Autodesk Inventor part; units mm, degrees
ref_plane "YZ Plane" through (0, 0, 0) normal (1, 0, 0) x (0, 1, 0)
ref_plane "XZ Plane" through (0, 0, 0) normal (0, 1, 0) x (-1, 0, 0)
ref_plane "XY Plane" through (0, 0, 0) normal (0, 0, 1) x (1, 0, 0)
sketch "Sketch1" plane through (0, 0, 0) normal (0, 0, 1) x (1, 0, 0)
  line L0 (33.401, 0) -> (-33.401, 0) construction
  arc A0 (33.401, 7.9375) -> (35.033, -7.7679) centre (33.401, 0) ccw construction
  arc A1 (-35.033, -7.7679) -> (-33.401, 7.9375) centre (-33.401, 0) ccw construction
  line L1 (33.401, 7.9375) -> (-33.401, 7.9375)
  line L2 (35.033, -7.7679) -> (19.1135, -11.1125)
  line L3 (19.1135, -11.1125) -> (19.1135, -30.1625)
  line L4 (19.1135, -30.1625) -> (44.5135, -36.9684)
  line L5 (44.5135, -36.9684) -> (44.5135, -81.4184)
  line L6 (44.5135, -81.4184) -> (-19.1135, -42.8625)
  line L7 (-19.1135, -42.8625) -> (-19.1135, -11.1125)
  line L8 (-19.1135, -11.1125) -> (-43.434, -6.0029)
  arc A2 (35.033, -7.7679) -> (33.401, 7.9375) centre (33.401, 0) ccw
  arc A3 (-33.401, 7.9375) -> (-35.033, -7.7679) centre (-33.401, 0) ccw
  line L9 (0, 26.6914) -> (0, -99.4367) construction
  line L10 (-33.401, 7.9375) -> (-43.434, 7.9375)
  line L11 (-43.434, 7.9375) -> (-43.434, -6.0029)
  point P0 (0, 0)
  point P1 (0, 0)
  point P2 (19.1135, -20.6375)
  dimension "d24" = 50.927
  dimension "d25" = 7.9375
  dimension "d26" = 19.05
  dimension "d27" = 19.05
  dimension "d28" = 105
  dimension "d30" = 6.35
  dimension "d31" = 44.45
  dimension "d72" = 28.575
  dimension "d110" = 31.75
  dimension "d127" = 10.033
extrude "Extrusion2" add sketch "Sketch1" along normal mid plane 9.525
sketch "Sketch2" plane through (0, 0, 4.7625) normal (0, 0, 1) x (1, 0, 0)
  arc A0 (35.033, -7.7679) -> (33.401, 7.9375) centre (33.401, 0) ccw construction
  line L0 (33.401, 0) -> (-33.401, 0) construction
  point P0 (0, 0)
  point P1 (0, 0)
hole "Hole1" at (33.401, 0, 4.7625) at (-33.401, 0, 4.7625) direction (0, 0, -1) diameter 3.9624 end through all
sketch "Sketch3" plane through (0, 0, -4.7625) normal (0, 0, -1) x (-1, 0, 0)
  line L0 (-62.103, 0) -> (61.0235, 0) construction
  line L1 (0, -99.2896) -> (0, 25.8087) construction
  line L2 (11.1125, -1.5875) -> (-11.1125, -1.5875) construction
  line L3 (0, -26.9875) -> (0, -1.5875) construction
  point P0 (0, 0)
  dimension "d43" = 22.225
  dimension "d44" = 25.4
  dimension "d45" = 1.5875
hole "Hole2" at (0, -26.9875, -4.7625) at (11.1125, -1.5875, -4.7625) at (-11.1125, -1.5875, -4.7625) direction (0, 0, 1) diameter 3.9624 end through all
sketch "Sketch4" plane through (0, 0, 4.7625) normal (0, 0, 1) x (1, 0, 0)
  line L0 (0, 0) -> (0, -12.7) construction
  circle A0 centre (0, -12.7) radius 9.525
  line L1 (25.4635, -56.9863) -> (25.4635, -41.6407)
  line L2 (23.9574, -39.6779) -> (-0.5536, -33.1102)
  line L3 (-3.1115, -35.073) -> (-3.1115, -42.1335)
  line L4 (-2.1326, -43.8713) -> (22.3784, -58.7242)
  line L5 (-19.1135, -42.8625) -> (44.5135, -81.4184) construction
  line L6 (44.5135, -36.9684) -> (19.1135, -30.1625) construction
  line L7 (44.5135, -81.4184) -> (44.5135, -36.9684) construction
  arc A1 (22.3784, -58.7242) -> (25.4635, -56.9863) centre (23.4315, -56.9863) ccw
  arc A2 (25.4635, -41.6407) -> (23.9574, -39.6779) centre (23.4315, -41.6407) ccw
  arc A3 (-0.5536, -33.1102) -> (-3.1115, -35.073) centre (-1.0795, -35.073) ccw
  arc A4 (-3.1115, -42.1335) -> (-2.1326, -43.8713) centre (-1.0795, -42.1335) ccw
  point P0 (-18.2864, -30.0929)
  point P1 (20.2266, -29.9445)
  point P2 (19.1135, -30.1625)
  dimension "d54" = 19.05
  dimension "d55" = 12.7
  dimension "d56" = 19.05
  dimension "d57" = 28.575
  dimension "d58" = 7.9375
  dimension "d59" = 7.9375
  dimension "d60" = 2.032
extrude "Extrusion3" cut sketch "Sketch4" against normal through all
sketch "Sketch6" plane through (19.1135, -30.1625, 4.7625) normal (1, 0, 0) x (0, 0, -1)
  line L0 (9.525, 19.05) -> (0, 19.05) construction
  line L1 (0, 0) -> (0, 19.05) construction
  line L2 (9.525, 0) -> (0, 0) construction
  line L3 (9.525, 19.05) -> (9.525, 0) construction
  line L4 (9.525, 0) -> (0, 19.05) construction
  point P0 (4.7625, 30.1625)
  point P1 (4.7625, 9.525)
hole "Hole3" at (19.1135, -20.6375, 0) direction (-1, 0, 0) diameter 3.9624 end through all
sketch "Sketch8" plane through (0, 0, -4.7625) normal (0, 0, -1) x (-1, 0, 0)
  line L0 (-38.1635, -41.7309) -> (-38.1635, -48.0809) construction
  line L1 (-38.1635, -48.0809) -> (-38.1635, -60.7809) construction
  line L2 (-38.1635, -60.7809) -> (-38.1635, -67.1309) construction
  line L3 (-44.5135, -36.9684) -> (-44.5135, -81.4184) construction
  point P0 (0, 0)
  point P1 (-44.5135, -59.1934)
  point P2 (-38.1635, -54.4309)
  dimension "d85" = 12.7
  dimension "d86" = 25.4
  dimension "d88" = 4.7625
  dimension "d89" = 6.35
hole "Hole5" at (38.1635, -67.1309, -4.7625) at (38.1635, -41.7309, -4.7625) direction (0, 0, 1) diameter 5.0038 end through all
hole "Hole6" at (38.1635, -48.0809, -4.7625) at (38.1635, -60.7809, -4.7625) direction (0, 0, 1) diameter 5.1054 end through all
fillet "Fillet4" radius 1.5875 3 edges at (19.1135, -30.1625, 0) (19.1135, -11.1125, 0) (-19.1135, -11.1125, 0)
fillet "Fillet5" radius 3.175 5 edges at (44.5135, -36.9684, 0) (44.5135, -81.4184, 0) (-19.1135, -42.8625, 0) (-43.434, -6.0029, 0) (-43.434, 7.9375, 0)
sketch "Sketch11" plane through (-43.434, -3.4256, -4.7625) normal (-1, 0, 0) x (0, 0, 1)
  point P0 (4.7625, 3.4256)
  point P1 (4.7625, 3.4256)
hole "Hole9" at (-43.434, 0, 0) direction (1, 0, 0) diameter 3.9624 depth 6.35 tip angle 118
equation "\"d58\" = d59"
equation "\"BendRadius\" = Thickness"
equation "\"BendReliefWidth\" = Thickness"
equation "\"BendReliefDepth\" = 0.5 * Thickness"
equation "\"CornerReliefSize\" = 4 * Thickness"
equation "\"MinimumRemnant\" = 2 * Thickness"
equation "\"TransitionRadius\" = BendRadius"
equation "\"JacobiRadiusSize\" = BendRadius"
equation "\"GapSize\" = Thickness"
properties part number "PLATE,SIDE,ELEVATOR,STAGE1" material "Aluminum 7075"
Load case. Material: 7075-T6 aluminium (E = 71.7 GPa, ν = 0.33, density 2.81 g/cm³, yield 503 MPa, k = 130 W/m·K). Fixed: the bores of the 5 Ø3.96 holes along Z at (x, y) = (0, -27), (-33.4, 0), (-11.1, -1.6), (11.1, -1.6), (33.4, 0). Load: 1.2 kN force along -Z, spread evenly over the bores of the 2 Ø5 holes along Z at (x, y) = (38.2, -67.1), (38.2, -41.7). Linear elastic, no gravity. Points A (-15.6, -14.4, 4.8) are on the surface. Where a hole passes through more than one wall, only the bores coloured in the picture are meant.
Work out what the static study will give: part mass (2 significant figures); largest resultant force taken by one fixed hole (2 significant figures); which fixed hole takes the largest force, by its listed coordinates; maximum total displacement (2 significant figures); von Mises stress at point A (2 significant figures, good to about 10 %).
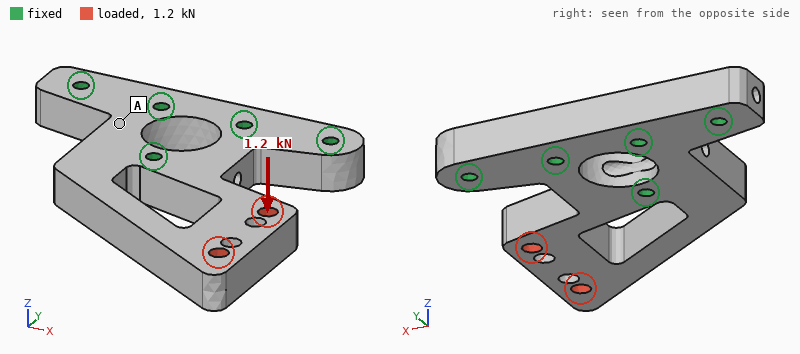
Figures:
86 g
1.7 kN
(0, -27)
0.79 mm
21 MPa
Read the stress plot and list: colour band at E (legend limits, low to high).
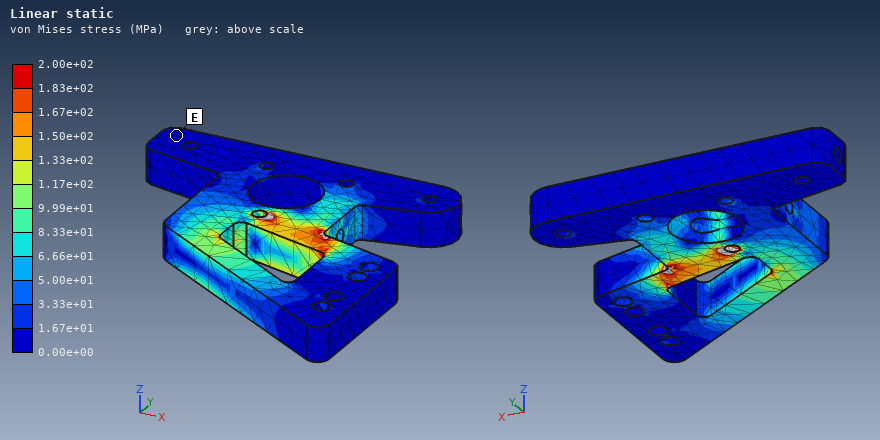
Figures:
0.00e+00 to 1.67e+01 MPa
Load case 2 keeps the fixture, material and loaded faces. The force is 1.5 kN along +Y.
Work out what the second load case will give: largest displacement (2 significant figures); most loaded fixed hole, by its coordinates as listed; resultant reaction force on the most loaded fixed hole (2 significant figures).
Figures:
0.11 mm
(11.1, -1.6)
1.8 kN
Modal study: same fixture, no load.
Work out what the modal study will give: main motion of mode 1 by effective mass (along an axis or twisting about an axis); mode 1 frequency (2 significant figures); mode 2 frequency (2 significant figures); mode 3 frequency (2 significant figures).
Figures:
along Z
1700 Hz
4100 Hz
5200 Hz
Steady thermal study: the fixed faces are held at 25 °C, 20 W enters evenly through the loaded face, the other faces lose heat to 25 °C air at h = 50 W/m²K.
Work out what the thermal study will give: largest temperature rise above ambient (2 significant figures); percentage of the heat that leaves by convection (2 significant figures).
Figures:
33 K
28 %
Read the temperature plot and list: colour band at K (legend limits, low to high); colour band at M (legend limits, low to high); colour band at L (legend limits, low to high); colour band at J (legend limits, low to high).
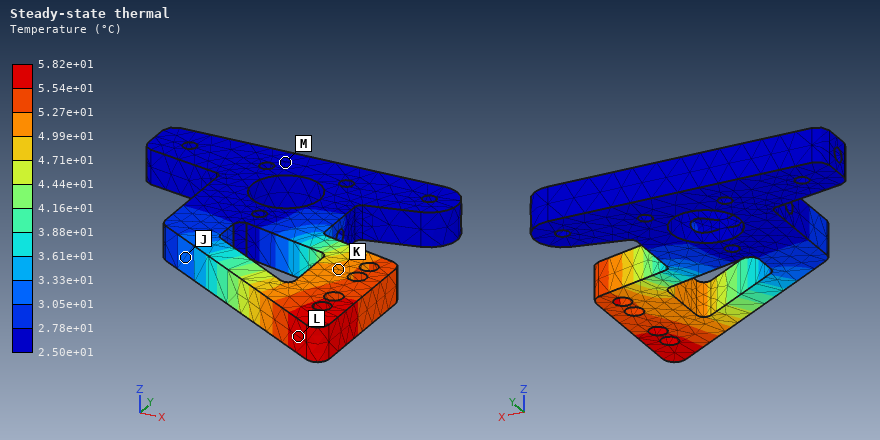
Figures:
4.99e+01 to 5.27e+01 °C
2.50e+01 to 2.78e+01 °C
5.54e+01 to 5.82e+01 °C
3.05e+01 to 3.33e+01 °C
